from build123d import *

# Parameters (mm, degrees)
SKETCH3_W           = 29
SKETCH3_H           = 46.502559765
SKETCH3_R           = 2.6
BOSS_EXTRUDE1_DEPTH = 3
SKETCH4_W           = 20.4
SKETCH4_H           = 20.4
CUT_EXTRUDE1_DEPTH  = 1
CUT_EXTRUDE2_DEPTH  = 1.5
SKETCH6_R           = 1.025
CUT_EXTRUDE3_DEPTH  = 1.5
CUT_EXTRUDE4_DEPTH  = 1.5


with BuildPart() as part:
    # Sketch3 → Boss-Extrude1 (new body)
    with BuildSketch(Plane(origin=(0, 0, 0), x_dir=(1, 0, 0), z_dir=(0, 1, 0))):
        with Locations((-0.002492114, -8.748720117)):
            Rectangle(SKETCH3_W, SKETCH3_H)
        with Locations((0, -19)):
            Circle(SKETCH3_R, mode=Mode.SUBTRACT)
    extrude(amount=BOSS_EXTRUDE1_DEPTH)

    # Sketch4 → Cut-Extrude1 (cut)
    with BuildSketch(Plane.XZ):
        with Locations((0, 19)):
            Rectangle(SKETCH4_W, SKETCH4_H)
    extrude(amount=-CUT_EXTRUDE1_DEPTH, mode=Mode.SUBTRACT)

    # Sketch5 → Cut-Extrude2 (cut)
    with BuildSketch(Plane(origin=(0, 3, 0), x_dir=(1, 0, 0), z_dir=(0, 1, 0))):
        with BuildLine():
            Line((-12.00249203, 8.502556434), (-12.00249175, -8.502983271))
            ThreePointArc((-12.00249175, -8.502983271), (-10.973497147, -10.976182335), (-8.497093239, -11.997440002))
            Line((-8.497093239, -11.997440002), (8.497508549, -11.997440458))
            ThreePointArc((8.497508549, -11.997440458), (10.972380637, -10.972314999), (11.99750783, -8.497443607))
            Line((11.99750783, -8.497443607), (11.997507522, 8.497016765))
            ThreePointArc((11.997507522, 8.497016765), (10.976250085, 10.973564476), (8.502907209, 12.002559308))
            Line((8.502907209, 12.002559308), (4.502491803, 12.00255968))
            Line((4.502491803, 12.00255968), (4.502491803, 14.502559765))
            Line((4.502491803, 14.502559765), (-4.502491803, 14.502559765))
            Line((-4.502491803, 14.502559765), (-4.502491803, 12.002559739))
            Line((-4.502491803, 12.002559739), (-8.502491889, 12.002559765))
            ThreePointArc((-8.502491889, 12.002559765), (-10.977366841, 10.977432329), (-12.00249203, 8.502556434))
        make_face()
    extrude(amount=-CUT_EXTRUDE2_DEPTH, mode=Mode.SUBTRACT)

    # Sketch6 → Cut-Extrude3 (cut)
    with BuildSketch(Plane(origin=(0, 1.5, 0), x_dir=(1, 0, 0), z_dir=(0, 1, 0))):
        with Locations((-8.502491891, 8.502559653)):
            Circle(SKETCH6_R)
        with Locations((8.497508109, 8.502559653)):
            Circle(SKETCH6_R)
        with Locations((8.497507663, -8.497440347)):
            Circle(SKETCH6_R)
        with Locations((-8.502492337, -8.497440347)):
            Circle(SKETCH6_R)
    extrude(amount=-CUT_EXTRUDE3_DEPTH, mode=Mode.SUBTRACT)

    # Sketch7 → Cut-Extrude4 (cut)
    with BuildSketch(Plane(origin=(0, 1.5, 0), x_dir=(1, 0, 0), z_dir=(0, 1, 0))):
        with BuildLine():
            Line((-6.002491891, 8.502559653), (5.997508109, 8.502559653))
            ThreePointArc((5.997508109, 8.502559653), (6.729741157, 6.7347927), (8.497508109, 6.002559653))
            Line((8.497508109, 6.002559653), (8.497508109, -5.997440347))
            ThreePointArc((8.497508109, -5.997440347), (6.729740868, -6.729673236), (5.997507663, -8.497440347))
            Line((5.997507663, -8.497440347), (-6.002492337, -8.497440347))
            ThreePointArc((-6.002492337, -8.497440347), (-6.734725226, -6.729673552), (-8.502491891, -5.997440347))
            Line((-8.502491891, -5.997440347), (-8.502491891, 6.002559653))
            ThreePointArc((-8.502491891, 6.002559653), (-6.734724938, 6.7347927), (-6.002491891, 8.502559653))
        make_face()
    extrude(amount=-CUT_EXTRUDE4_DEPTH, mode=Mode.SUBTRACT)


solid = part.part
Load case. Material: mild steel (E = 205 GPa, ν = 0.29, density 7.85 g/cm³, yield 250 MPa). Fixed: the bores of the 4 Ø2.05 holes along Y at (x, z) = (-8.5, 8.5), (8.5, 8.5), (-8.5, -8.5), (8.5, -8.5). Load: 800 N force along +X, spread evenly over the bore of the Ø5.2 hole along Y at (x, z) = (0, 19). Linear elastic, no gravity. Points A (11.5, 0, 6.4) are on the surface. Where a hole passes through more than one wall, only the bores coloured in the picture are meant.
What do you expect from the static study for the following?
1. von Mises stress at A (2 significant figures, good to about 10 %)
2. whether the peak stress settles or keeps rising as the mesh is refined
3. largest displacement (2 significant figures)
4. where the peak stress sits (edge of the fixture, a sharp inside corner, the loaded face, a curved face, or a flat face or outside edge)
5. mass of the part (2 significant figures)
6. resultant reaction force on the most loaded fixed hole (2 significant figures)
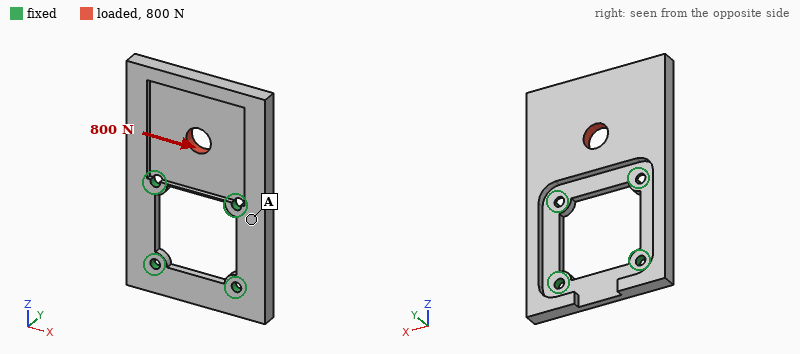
22 MPa
keeps rising
8.4 µm
edge of the fixture
18 g
500 N
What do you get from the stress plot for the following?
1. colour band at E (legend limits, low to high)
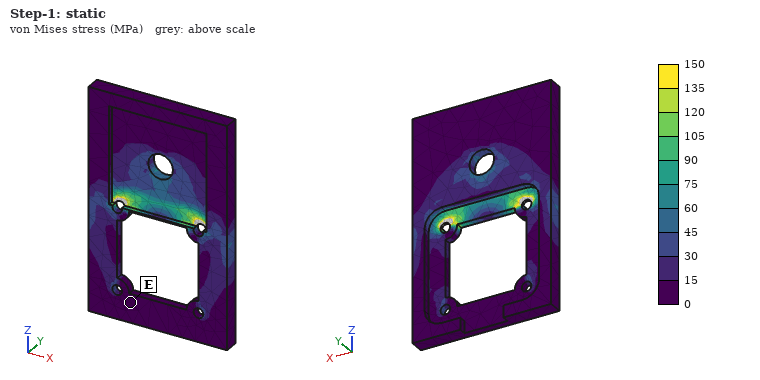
0 to 15 MPa
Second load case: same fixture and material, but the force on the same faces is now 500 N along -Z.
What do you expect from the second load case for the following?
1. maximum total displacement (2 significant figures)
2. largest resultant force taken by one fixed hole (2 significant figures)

27 µm
210 N
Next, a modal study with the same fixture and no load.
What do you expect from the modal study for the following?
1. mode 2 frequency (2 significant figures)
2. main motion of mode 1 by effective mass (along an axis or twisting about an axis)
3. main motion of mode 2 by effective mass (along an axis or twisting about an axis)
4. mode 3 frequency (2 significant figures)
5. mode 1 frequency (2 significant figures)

4900 Hz
along Y
twisting about Z
14 kHz
1900 Hz
